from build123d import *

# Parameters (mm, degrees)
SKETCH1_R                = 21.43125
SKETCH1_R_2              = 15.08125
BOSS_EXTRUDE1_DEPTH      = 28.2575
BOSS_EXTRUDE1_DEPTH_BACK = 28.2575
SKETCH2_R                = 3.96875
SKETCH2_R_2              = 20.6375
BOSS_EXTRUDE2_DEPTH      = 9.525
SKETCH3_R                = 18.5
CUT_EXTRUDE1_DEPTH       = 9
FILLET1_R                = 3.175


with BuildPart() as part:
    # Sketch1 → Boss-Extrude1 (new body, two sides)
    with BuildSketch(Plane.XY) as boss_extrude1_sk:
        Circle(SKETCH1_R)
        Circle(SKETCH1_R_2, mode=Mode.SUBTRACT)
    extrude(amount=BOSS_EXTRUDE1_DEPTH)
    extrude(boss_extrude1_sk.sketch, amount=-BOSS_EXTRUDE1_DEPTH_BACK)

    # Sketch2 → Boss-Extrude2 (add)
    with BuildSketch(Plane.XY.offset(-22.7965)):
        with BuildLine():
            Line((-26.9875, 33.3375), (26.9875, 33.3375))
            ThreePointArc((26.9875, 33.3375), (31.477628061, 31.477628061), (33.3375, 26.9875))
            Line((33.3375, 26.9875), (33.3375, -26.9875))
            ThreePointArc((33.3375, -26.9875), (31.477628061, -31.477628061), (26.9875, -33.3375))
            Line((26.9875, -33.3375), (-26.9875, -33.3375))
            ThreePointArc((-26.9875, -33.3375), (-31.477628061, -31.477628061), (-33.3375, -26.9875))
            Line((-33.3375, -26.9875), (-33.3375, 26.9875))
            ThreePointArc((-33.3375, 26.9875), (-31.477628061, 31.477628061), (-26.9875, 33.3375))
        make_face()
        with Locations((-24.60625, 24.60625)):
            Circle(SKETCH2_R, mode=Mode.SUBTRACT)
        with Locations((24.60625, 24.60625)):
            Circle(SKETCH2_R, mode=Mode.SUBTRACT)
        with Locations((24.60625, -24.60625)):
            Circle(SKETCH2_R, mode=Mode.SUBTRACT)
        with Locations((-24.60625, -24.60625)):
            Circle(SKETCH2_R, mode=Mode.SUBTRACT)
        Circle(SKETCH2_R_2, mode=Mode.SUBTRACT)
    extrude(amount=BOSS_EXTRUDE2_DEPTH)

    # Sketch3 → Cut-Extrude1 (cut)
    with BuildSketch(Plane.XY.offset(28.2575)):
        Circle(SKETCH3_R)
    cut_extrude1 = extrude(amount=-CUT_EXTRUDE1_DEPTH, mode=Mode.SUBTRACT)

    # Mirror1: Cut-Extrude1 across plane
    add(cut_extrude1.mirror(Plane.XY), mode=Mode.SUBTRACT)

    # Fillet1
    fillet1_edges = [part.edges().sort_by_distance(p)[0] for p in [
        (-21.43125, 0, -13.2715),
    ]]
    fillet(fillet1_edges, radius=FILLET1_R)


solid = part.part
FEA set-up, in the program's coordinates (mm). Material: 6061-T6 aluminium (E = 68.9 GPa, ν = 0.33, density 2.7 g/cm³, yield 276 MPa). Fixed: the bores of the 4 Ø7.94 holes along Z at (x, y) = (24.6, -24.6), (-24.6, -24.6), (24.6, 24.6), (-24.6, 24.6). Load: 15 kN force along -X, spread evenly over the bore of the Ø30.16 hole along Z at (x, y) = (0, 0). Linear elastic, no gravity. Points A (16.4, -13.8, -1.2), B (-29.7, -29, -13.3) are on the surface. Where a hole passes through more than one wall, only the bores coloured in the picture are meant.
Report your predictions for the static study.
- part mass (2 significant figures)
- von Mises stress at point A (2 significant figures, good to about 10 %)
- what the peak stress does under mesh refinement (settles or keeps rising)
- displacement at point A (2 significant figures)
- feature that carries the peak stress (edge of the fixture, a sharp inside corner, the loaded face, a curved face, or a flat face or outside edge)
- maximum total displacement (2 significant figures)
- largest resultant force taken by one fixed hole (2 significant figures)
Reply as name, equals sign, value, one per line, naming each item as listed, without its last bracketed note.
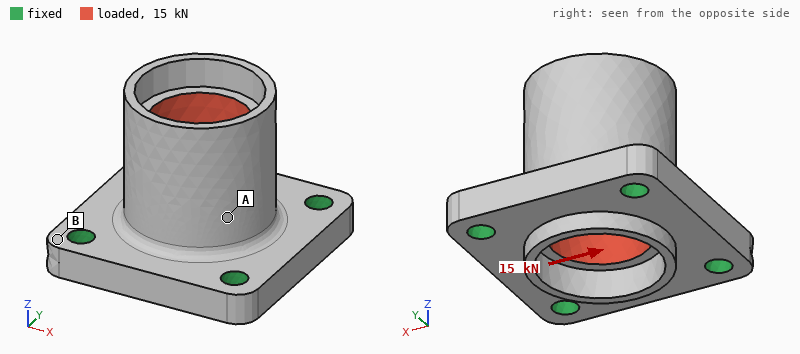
part mass = 170 g
von Mises stress at point A = 18 MPa
what the peak stress does under mesh refinement = keeps rising
displacement at point A = 33 µm
feature that carries the peak stress = edge of the fixture
maximum total displacement = 69 µm
largest resultant force taken by one fixed hole = 5.0 kN
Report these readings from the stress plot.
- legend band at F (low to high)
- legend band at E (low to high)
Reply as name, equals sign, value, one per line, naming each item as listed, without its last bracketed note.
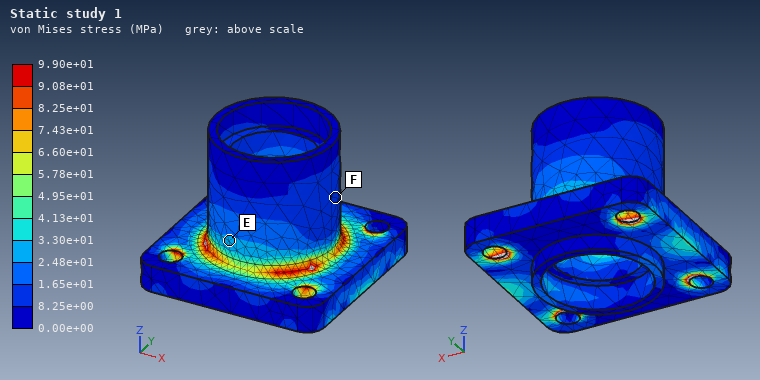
legend band at F = 8.25e+00 to 1.65e+01 MPa
legend band at E = 2.48e+01 to 3.30e+01 MPa
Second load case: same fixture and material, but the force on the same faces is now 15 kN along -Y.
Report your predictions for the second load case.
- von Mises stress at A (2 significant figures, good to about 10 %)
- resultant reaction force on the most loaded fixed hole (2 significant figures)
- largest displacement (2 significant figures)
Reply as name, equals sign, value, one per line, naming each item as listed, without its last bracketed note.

von Mises stress at A = 20 MPa
resultant reaction force on the most loaded fixed hole = 5.0 kN
largest displacement = 69 µm
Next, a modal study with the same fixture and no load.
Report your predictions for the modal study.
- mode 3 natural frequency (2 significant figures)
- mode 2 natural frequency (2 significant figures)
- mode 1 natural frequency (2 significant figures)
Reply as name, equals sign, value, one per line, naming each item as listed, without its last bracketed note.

mode 3 natural frequency = 12 kHz
mode 2 natural frequency = 8300 Hz
mode 1 natural frequency = 8300 Hz
